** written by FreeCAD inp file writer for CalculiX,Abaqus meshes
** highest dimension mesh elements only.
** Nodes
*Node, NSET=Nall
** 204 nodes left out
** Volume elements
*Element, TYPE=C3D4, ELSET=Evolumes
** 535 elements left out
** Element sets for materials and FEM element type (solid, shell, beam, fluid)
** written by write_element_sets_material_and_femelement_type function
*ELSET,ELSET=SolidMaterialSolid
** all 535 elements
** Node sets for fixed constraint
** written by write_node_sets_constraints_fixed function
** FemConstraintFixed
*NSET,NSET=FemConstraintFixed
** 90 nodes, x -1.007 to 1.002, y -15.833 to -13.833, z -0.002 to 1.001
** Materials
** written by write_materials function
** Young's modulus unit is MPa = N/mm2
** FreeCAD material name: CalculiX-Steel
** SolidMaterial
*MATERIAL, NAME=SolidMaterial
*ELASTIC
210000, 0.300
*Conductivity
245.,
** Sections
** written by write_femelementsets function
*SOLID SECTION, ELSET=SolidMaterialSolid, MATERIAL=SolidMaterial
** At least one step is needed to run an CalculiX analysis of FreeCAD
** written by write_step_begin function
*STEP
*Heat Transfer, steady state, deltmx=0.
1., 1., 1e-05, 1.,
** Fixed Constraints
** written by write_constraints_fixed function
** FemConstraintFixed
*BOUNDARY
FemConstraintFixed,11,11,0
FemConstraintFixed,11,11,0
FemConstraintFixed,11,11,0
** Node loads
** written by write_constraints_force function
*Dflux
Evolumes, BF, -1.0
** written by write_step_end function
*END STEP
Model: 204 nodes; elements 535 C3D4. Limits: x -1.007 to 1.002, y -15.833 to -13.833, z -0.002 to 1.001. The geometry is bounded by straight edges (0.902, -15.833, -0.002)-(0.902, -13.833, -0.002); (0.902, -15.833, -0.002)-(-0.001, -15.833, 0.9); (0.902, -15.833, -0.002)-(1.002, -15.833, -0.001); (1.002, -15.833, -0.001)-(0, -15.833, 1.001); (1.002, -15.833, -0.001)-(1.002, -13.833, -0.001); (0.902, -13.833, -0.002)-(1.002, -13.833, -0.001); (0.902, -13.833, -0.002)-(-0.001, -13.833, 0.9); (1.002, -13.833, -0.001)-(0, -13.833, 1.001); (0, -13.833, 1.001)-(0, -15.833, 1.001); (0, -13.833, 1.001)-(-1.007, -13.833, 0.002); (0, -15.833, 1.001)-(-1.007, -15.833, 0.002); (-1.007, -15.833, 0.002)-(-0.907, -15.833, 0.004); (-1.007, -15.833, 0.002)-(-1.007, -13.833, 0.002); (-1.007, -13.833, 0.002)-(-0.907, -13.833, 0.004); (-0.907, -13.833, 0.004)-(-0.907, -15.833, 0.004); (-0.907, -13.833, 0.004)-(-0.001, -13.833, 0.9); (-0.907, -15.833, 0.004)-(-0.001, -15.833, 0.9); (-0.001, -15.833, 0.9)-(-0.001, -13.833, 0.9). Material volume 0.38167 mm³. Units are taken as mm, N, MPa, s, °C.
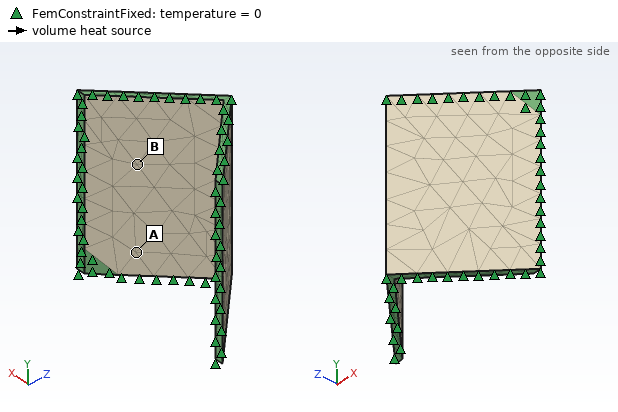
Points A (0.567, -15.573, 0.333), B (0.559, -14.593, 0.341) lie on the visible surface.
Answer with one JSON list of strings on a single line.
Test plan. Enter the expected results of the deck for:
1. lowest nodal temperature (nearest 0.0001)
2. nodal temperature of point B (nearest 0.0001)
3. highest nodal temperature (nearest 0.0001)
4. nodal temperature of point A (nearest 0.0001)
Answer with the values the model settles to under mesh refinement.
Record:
["-0.0015 °C", "-0.0010 °C", "0.0000 °C", "-0.0005 °C"]
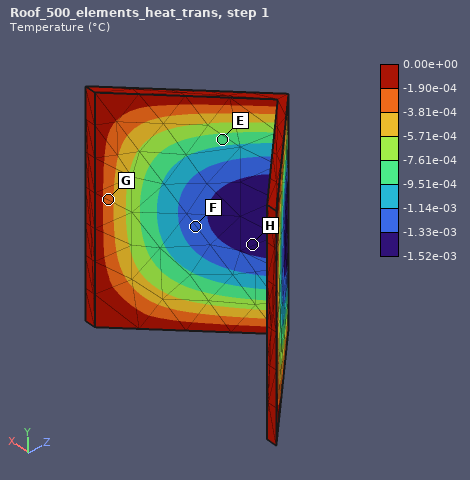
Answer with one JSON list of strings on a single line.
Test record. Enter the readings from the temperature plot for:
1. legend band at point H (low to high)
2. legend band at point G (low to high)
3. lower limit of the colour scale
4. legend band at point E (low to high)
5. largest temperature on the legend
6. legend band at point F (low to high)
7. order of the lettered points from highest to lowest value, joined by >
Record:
["-1.52e-03 to -1.33e-03 °C", "-3.81e-04 to -1.90e-04 °C", "-1.52e-03 °C", "-9.51e-04 to -7.61e-04 °C", "0.00e+00 °C", "-1.33e-03 to -1.14e-03 °C", "G > E > F > H"]
